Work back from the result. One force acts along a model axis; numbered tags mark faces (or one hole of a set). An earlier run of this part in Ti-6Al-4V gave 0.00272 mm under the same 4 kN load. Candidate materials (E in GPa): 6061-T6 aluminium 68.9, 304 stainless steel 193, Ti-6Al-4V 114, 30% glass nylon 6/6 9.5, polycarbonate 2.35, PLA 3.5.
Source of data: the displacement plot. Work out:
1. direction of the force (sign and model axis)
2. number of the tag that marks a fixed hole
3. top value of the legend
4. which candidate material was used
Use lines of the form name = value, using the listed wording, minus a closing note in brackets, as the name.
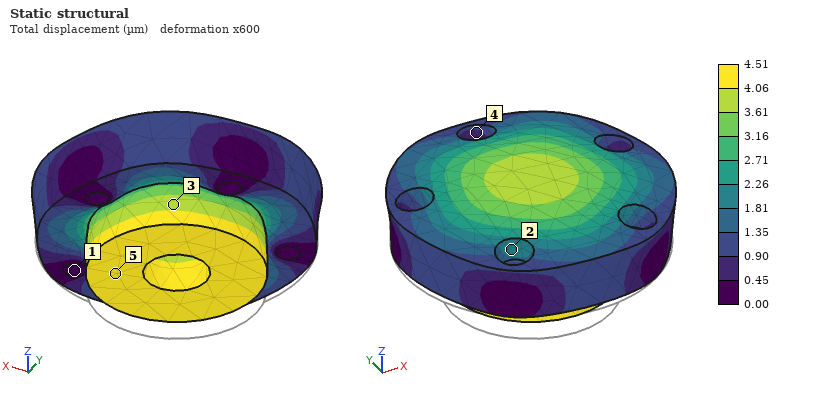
direction of the force = +Z
number of the tag that marks a fixed hole = 1
top value of the legend = 4.51 µm
which candidate material was used = 6061-T6 aluminium
